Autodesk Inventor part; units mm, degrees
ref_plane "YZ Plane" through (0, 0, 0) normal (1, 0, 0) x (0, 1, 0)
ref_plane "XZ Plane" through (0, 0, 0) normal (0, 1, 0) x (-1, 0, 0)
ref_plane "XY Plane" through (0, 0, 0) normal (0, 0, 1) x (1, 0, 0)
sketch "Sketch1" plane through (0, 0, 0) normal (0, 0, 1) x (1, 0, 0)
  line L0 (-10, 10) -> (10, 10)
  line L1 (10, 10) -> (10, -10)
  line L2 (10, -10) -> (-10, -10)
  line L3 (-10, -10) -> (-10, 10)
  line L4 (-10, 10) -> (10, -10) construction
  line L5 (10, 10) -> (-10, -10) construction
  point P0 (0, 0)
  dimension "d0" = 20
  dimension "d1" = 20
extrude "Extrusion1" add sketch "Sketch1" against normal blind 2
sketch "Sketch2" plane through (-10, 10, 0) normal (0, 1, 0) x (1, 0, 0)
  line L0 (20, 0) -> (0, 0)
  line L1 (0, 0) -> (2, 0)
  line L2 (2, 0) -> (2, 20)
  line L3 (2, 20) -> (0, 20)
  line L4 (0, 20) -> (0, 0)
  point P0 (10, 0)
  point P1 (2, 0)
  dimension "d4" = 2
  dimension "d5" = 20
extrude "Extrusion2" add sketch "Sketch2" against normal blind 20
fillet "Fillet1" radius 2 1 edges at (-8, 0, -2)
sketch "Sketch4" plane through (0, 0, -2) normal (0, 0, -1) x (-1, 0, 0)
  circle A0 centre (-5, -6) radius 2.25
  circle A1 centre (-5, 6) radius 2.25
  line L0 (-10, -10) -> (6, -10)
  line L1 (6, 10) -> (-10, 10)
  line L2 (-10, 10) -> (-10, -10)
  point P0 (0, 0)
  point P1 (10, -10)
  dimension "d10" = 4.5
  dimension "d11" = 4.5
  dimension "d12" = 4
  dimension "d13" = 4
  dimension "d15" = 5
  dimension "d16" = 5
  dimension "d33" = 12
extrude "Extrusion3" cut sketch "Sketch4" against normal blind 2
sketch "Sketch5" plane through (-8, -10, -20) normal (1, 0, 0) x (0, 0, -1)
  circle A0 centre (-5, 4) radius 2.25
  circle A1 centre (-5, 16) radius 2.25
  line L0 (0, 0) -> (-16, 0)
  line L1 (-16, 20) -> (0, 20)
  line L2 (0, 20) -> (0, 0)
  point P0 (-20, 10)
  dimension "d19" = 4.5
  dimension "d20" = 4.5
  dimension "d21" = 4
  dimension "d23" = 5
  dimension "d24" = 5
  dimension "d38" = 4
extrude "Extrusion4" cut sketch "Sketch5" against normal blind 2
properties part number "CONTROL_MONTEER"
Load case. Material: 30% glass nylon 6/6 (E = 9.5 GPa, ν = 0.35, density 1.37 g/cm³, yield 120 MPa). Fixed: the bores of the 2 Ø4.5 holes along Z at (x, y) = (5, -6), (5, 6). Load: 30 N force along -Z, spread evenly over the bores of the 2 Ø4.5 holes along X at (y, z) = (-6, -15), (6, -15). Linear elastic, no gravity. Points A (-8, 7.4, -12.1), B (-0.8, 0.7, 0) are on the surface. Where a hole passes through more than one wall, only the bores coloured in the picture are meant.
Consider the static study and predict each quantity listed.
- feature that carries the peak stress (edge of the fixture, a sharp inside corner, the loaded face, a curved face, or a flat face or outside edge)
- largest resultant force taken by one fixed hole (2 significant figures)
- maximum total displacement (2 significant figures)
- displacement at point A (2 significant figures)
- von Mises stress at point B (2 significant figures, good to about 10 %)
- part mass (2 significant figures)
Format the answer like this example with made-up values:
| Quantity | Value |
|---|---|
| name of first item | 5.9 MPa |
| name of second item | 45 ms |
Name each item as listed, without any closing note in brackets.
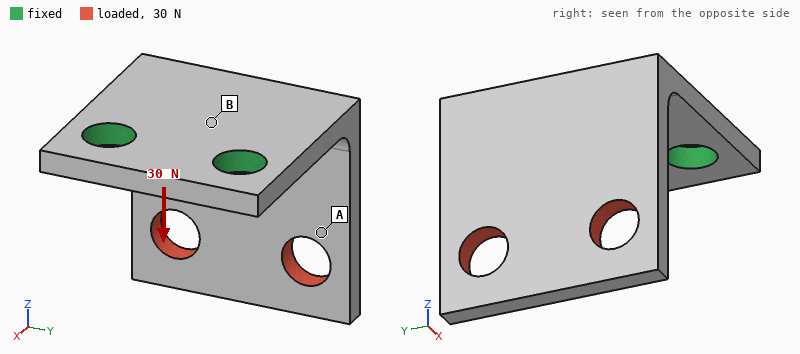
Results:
| Quantity | Value |
|---|---|
| feature that carries the peak stress | a flat face or outside edge |
| largest resultant force taken by one fixed hole | 15 N |
| maximum total displacement | 0.36 mm |
| displacement at point A | 0.23 mm |
| von Mises stress at point B | 15 MPa |
| part mass | 1.9 g |
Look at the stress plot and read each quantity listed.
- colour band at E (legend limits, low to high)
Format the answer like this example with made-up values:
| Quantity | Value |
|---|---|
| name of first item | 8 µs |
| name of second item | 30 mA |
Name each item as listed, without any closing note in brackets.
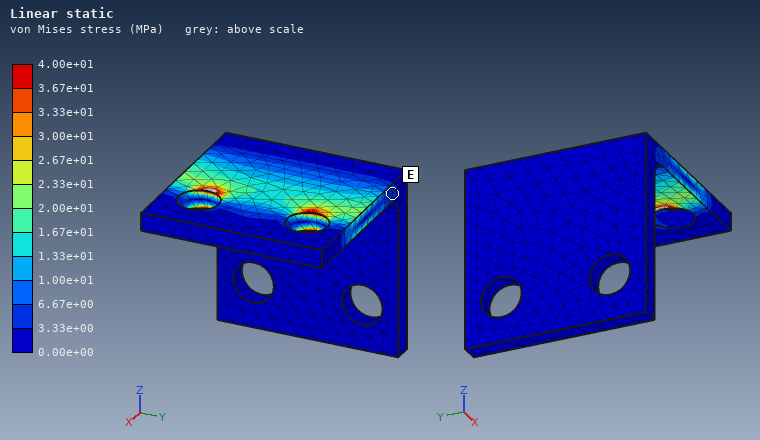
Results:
| Quantity | Value |
|---|---|
| colour band at E | 3.33e+00 to 6.67e+00 MPa |
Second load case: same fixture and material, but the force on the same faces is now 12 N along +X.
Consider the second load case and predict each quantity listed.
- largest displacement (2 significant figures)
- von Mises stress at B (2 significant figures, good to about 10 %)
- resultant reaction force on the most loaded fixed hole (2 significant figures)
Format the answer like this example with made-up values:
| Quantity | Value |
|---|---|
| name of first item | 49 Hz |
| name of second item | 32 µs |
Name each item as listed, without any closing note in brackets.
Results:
| Quantity | Value |
|---|---|
| largest displacement | 0.38 mm |
| von Mises stress at B | 10 MPa |
| resultant reaction force on the most loaded fixed hole | 6.4 N |
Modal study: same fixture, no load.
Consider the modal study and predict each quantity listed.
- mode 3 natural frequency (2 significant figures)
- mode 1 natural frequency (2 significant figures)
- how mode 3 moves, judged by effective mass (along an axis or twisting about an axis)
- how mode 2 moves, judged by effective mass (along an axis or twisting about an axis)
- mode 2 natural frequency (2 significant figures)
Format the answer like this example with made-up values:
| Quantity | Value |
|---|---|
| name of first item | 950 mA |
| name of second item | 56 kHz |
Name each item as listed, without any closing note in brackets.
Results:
| Quantity | Value |
|---|---|
| mode 3 natural frequency | 3800 Hz |
| mode 1 natural frequency | 1300 Hz |
| how mode 3 moves, judged by effective mass | along Z |
| how mode 2 moves, judged by effective mass | along Y |
| mode 2 natural frequency | 2400 Hz |
